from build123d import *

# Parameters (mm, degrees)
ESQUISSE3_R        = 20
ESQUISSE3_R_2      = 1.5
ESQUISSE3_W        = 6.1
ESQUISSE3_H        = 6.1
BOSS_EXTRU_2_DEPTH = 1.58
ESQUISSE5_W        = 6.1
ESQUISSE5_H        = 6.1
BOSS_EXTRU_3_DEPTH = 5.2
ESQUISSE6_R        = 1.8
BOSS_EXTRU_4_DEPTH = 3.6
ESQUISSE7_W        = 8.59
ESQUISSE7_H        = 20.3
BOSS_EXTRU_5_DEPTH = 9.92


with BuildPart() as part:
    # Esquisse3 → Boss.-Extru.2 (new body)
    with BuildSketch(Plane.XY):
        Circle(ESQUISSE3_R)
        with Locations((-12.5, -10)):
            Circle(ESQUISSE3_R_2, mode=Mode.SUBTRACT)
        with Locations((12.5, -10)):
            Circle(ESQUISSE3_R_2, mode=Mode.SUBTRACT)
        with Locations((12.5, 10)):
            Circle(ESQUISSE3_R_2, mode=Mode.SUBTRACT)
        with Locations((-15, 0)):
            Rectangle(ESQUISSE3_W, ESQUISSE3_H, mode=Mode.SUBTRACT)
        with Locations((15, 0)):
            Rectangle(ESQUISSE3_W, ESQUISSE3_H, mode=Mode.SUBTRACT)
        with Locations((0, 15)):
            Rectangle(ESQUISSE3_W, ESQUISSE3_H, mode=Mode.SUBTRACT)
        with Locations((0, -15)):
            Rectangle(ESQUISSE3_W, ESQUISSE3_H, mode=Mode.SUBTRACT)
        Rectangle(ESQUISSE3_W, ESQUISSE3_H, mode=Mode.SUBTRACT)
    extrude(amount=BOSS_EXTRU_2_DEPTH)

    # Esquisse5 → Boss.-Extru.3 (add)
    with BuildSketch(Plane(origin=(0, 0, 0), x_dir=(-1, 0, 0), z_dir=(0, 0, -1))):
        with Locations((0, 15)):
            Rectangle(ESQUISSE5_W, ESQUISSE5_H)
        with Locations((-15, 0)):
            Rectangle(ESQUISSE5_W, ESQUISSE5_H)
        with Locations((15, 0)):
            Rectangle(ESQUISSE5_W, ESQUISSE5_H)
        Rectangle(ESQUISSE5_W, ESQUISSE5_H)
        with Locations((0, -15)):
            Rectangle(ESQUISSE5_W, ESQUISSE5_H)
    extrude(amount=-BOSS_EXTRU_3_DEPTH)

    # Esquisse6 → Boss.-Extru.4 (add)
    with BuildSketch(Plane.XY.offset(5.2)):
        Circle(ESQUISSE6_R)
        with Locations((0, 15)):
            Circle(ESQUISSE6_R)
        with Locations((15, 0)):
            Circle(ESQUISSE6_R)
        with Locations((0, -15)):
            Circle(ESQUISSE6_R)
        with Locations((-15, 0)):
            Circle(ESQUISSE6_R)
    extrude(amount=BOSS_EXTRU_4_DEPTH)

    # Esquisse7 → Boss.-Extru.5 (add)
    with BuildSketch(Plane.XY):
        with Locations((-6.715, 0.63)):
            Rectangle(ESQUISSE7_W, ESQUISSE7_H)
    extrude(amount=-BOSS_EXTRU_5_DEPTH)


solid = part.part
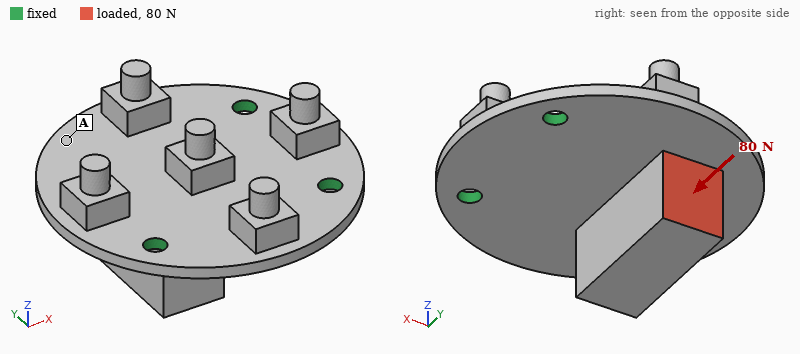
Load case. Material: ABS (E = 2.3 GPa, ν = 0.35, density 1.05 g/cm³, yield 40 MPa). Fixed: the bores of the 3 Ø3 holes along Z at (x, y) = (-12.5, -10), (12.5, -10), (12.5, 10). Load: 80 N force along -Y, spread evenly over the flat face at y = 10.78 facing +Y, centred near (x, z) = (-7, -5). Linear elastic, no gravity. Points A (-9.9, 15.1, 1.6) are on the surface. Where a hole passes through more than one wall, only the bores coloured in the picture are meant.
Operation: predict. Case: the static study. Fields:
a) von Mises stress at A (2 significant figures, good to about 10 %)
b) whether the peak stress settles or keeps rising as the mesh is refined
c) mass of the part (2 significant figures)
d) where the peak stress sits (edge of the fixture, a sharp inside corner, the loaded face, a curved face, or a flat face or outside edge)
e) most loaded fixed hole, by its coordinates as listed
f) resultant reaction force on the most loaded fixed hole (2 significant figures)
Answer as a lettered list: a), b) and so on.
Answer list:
a) 4.0 MPa
b) keeps rising
c) 4.8 g
d) edge of the fixture
e) (-12.5, -10)
f) 58 N
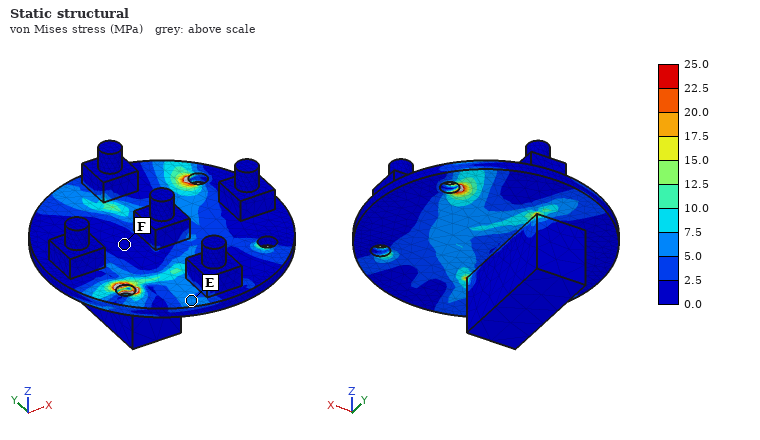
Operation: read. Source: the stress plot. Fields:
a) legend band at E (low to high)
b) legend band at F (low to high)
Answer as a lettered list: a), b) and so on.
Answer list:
a) 5.0 to 7.5 MPa
b) 0.0 to 2.5 MPa
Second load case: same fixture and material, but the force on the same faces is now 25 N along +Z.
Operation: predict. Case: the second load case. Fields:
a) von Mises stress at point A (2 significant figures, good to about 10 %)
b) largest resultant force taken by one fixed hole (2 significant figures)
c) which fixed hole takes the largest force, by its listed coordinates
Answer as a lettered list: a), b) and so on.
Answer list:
a) 3.6 MPa
b) 17 N
c) (12.5, 10)
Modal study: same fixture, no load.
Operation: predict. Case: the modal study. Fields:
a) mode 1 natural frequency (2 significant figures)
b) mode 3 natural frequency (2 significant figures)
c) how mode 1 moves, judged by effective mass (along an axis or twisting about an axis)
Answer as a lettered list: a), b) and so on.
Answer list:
a) 940 Hz
b) 2800 Hz
c) along Z
